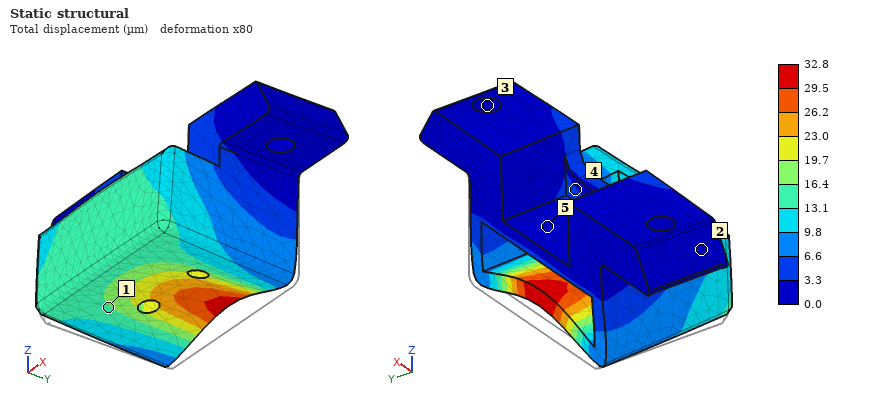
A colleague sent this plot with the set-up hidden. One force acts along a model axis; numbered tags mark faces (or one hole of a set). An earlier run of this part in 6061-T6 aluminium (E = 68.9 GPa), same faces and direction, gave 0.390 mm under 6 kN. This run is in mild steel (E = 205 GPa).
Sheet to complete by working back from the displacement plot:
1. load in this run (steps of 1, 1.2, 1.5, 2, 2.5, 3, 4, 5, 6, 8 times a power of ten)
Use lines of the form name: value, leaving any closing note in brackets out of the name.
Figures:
load in this run: 1.5 kN
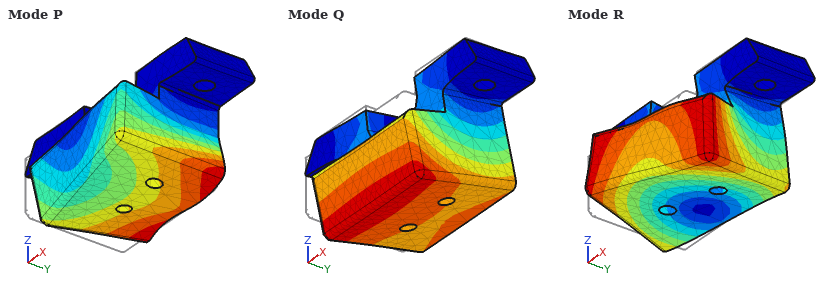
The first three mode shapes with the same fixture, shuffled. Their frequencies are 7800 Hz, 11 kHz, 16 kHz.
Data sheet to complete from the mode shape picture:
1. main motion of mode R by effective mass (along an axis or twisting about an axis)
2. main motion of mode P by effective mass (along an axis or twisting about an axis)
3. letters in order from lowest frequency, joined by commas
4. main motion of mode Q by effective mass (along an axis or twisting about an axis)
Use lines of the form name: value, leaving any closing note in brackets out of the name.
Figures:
main motion of mode R by effective mass: along X
main motion of mode P by effective mass: along X
letters in order from lowest frequency, joined by commas: Q, P, R
main motion of mode Q by effective mass: along Y
